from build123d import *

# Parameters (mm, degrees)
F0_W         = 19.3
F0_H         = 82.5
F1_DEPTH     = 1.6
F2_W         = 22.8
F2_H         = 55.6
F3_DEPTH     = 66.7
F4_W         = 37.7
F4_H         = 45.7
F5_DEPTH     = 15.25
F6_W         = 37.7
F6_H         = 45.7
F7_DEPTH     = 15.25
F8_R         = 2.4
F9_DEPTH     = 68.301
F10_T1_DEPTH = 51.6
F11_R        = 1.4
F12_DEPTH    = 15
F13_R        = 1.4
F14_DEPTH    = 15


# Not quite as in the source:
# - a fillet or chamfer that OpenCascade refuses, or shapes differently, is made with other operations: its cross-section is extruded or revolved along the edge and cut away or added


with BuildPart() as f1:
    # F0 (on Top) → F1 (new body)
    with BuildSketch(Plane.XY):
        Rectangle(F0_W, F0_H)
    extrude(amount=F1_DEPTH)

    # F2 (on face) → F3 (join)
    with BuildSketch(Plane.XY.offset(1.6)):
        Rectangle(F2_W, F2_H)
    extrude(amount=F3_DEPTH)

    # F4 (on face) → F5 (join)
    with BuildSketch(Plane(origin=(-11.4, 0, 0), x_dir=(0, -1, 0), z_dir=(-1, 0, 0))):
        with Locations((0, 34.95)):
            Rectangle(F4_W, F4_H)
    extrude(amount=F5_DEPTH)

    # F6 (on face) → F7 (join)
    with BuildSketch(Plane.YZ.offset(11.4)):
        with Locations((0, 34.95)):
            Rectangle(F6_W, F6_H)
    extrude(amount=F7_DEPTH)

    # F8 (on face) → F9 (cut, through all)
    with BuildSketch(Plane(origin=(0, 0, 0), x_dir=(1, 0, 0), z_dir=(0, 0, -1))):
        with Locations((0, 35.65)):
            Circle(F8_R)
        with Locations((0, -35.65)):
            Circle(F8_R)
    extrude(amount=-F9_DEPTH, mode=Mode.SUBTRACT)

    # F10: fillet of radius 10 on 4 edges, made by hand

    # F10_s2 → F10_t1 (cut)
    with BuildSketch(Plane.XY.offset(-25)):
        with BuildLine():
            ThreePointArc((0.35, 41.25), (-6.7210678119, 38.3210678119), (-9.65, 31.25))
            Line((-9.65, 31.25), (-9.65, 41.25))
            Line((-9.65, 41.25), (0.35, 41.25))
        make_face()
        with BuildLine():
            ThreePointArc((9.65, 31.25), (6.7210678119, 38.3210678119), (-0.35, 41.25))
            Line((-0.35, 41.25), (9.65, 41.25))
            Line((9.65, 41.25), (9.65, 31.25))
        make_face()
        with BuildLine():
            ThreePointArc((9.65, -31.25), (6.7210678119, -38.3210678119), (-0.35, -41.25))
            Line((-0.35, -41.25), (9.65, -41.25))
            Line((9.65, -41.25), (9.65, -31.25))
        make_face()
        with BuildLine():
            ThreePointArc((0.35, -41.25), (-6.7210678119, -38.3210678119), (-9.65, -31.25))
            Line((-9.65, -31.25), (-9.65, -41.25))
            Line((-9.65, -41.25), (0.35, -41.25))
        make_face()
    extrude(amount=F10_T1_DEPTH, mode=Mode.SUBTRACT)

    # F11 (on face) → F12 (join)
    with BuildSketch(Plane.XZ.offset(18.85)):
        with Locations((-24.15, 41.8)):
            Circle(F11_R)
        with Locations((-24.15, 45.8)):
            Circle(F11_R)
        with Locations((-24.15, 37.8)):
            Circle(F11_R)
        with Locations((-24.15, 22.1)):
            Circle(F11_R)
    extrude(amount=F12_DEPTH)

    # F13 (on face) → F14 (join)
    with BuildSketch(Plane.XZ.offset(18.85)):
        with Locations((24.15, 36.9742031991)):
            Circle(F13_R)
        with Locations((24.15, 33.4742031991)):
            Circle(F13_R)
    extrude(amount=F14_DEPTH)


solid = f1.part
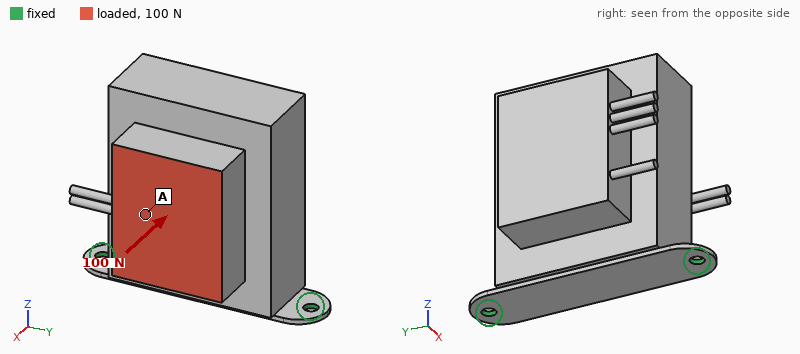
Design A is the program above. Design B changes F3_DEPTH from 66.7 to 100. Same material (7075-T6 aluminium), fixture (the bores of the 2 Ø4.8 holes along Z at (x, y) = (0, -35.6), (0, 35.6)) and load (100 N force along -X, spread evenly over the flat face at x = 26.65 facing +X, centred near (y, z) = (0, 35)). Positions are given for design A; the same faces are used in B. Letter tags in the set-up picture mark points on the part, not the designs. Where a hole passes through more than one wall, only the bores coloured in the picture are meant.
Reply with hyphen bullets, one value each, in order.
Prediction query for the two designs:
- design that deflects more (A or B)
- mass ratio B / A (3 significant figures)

- B
- 1.30
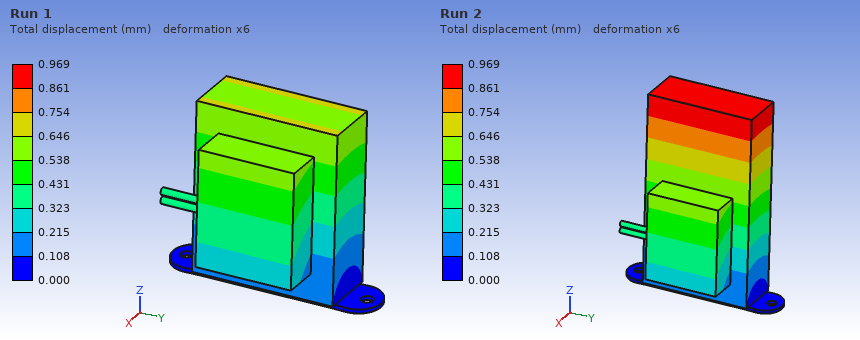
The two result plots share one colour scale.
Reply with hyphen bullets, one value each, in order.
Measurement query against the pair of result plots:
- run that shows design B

- Run 2
